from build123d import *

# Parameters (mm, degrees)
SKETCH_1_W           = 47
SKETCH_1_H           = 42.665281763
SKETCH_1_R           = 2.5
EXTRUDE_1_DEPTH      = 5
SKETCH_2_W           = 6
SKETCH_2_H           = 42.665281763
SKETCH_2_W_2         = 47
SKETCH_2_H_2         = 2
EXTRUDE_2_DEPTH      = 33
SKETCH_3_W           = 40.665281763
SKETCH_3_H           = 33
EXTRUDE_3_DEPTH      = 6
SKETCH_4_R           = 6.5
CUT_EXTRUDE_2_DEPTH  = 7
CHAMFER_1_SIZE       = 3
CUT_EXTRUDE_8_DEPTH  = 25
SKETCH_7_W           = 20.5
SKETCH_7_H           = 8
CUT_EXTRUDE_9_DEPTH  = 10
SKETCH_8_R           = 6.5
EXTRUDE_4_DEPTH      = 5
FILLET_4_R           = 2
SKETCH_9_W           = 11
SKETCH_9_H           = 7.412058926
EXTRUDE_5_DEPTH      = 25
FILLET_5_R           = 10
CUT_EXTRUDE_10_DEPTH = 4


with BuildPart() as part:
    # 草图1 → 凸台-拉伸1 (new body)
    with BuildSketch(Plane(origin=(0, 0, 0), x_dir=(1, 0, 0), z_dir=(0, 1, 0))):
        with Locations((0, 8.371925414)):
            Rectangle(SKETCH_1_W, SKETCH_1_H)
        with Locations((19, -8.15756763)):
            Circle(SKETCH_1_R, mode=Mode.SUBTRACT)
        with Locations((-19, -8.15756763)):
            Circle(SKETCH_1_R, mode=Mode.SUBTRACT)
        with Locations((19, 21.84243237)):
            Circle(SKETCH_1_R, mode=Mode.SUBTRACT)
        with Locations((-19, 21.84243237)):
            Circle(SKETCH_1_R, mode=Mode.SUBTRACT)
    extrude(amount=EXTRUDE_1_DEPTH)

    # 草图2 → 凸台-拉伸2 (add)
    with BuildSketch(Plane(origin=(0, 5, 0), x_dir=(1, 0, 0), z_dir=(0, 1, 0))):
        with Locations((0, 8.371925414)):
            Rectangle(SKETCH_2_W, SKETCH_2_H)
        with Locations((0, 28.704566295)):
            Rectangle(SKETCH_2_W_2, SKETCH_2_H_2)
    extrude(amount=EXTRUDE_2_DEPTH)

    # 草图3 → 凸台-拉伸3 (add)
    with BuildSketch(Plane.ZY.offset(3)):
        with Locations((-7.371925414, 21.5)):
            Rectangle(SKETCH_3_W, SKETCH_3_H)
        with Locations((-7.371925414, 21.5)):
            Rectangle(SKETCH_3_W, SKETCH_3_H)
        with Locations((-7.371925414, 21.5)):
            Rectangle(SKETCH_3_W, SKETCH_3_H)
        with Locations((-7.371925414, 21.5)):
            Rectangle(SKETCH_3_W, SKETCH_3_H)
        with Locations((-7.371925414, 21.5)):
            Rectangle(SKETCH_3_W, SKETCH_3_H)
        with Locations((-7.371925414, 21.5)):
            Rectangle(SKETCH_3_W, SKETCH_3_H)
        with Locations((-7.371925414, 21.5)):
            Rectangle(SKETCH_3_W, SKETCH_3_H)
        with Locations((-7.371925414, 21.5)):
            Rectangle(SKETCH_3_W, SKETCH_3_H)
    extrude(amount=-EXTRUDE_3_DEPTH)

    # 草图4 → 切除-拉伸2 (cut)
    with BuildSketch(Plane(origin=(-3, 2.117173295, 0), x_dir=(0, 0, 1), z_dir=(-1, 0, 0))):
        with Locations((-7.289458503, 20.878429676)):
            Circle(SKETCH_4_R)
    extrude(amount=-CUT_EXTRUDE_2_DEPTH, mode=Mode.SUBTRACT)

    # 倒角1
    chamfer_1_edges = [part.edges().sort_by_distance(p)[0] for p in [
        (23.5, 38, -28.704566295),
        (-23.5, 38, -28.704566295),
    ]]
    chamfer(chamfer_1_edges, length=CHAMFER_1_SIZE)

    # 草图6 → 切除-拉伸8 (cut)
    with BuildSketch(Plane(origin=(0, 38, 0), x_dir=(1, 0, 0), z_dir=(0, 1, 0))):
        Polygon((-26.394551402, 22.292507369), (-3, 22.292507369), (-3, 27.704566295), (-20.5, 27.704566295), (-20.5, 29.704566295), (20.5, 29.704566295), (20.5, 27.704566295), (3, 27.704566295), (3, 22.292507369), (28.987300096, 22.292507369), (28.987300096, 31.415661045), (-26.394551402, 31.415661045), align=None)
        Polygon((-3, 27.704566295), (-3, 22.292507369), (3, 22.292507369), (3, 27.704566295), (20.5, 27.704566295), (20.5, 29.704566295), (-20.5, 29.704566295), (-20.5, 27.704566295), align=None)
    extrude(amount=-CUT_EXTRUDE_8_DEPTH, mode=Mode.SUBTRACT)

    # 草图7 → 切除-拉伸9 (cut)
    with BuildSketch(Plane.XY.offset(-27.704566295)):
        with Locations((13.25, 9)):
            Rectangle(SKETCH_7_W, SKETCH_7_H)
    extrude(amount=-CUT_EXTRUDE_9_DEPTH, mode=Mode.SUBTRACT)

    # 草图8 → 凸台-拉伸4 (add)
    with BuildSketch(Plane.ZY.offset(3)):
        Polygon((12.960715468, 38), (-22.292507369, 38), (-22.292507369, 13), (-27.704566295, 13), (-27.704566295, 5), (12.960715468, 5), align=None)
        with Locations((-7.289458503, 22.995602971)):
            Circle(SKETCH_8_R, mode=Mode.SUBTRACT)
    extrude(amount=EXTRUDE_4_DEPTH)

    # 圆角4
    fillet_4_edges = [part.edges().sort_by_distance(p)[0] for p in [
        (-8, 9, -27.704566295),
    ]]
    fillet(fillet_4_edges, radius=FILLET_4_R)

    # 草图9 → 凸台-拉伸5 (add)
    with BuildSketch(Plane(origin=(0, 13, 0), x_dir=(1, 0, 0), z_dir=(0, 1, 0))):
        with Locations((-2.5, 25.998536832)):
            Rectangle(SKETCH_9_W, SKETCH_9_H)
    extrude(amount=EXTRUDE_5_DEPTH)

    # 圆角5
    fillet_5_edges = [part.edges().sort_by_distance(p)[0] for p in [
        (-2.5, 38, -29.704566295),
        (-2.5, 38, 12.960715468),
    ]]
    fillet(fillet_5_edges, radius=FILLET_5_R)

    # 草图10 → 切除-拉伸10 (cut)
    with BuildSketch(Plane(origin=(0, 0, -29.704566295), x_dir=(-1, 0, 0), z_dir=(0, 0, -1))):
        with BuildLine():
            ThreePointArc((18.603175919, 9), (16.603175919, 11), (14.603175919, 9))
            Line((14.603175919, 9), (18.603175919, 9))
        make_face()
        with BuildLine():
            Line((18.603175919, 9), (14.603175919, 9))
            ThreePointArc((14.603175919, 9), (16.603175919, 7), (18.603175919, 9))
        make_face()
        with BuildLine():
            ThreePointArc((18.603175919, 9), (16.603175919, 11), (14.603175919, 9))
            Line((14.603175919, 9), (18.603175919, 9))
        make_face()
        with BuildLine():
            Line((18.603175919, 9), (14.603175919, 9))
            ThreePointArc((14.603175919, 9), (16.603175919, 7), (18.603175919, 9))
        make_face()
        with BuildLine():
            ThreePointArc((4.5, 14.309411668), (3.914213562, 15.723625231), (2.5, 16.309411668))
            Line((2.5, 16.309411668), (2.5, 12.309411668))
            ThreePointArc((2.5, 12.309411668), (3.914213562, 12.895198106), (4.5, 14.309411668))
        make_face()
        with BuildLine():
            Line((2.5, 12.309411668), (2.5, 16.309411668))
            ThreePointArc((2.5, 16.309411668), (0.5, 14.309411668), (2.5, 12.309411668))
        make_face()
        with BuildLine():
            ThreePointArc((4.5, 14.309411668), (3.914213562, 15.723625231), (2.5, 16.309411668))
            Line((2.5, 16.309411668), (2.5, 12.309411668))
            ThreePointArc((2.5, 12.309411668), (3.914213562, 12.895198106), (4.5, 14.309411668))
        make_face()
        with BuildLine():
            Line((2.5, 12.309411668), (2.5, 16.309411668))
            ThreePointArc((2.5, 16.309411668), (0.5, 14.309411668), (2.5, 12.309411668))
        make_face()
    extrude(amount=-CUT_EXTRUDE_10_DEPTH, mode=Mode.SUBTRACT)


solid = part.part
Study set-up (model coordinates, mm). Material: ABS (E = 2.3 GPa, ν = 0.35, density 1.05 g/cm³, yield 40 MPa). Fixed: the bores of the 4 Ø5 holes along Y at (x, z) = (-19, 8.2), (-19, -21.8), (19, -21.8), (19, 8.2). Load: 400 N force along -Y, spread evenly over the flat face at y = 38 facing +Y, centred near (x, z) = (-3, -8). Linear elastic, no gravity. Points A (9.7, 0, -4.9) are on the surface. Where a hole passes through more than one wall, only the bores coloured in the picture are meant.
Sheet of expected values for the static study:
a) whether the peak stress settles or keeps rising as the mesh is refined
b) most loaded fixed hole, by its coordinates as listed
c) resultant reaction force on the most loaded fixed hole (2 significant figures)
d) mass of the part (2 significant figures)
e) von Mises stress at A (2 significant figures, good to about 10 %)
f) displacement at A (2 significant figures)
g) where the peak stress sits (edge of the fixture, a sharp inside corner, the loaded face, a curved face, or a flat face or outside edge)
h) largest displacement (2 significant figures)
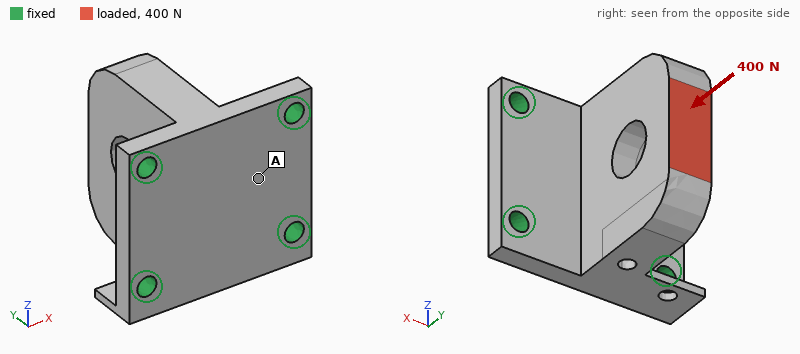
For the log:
keeps rising
(-19, -21.8)
130 N
25 g
1.7 MPa
0.061 mm
edge of the fixture
0.14 mm
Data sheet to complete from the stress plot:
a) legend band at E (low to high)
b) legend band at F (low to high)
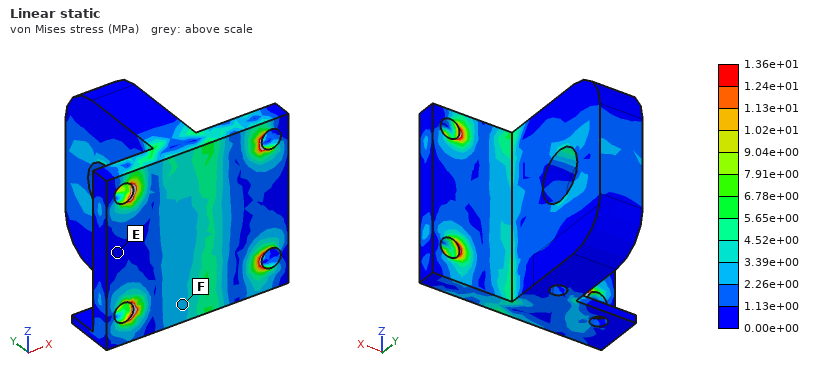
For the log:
0.00e+00 to 1.13e+00 MPa
2.26e+00 to 3.39e+00 MPa
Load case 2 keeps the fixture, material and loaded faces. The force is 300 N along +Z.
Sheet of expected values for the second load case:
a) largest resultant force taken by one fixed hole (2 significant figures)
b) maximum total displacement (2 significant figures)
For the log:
260 N
0.41 mm
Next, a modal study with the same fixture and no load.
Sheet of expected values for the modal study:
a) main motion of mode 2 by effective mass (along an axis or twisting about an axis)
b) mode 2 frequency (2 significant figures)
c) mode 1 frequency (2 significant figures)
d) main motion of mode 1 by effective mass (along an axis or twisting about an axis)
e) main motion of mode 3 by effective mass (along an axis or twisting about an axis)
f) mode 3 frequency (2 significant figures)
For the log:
along Z
1700 Hz
1400 Hz
along X
along Y
2700 Hz
